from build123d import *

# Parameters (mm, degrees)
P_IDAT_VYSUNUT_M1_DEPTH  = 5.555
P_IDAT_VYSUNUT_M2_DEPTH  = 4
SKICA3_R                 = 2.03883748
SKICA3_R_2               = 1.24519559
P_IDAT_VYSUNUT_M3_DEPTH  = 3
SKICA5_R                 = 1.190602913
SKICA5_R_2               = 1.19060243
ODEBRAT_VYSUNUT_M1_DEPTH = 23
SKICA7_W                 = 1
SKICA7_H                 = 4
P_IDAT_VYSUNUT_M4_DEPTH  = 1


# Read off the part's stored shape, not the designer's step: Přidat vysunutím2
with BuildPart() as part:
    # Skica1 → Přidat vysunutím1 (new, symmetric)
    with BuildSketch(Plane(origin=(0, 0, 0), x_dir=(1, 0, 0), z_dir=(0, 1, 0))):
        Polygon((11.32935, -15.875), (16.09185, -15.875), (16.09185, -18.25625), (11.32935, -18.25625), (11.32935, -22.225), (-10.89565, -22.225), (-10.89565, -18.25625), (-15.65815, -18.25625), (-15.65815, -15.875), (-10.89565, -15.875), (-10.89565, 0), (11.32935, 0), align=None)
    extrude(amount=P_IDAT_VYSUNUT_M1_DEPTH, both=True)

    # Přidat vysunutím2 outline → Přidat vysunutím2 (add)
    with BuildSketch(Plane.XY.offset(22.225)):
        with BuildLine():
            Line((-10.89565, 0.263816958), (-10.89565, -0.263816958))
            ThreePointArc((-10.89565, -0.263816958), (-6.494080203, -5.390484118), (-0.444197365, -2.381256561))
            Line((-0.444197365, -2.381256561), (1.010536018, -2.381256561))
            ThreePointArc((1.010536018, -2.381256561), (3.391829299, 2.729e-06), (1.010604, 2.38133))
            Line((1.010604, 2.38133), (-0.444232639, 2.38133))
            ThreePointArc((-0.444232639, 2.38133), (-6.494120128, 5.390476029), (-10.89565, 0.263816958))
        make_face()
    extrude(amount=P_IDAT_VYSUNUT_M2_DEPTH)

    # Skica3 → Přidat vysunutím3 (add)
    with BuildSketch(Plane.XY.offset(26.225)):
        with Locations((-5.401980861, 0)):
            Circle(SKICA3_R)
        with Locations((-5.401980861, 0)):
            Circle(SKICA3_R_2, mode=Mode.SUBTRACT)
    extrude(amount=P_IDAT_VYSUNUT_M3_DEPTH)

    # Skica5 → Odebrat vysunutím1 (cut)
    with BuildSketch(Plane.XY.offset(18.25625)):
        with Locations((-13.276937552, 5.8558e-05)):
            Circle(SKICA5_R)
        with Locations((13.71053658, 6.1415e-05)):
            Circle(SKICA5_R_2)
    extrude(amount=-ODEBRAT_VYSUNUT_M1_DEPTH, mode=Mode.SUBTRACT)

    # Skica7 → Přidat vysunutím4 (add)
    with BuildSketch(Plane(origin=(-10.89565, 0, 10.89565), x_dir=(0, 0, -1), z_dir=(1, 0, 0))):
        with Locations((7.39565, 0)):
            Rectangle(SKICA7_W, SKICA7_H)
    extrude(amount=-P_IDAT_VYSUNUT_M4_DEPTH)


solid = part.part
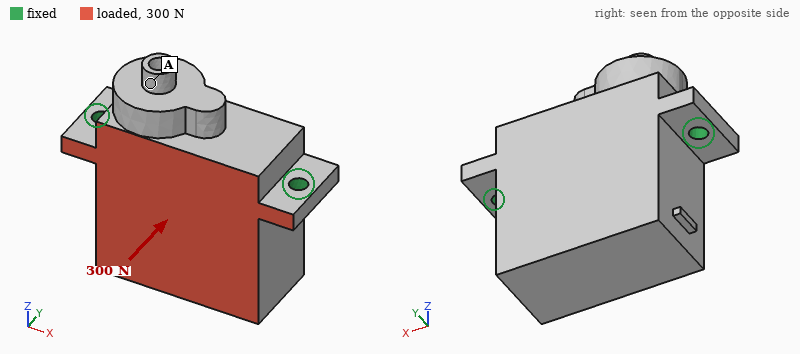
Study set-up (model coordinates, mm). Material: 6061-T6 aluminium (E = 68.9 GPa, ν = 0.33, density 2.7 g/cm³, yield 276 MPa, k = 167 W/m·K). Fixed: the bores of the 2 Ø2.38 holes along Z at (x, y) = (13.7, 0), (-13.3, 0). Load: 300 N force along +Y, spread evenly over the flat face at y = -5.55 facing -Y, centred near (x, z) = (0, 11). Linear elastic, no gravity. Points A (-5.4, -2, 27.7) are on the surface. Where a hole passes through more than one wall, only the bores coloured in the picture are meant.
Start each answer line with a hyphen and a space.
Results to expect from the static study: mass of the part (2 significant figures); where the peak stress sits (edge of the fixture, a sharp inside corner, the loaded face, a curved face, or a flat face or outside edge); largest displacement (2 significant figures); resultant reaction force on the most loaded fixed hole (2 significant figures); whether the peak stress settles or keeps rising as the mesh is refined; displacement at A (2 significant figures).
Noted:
- 17 g
- edge of the fixture
- 32 µm
- 150 N
- keeps rising
- 16 µm
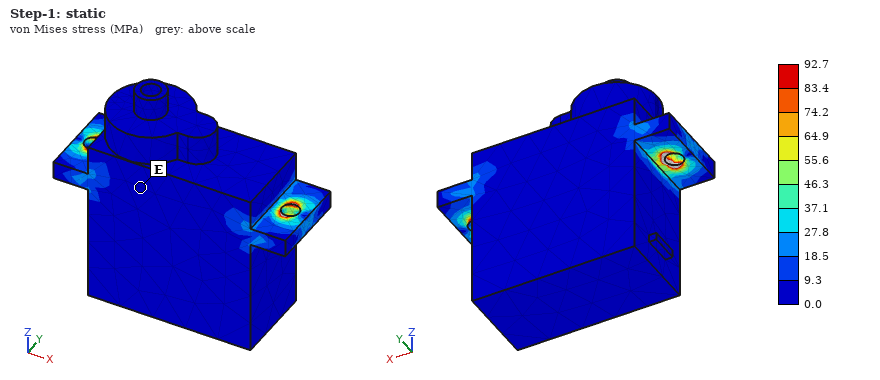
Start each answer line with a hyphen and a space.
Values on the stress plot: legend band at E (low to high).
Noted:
- 0.0 to 9.3 MPa
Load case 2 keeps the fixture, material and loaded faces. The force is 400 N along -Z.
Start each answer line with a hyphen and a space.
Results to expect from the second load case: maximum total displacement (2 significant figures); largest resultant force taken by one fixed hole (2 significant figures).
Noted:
- 40 µm
- 200 N
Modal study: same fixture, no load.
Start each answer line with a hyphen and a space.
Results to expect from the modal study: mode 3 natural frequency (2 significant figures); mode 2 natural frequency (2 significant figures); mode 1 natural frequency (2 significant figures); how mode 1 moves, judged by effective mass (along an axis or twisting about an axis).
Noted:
- 18 kHz
- 17 kHz
- 4300 Hz
- along Y
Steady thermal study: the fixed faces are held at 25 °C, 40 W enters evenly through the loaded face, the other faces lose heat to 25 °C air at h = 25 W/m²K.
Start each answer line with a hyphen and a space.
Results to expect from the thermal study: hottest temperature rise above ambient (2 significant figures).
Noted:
- 26 K
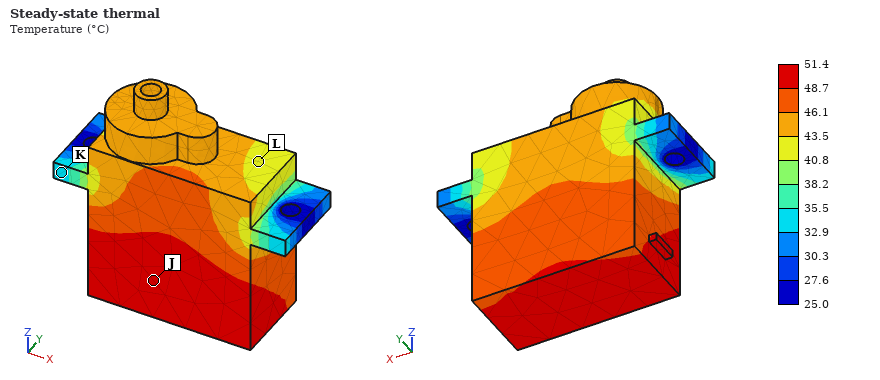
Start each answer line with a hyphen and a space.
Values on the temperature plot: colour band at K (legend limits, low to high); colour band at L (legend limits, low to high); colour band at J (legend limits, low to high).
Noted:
- 32.9 to 35.5 °C
- 40.8 to 43.5 °C
- 48.7 to 51.4 °C
